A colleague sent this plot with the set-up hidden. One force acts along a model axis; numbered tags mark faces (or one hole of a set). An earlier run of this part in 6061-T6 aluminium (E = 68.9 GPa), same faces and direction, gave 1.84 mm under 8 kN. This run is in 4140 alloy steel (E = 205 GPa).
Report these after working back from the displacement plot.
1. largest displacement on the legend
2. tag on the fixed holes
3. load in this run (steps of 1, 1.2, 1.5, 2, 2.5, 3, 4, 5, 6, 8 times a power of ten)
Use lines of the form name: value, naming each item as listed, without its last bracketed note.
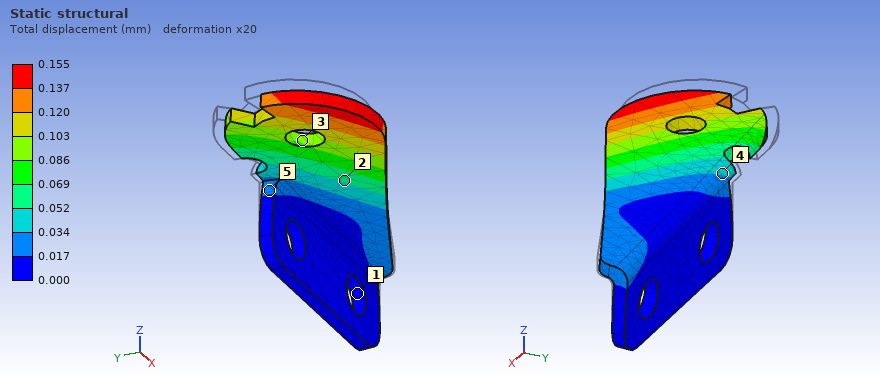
largest displacement on the legend: 0.155 mm
tag on the fixed holes: 1
load in this run: 2 kN
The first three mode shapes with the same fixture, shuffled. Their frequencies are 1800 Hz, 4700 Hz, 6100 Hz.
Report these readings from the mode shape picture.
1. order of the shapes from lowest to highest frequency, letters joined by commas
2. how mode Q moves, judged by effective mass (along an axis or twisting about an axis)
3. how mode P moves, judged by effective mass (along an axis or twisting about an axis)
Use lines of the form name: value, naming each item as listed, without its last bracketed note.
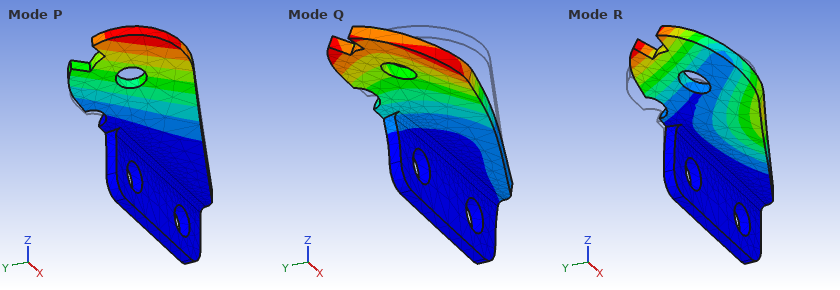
order of the shapes from lowest to highest frequency, letters joined by commas: P, R, Q
how mode Q moves, judged by effective mass: along Y
how mode P moves, judged by effective mass: along Z
